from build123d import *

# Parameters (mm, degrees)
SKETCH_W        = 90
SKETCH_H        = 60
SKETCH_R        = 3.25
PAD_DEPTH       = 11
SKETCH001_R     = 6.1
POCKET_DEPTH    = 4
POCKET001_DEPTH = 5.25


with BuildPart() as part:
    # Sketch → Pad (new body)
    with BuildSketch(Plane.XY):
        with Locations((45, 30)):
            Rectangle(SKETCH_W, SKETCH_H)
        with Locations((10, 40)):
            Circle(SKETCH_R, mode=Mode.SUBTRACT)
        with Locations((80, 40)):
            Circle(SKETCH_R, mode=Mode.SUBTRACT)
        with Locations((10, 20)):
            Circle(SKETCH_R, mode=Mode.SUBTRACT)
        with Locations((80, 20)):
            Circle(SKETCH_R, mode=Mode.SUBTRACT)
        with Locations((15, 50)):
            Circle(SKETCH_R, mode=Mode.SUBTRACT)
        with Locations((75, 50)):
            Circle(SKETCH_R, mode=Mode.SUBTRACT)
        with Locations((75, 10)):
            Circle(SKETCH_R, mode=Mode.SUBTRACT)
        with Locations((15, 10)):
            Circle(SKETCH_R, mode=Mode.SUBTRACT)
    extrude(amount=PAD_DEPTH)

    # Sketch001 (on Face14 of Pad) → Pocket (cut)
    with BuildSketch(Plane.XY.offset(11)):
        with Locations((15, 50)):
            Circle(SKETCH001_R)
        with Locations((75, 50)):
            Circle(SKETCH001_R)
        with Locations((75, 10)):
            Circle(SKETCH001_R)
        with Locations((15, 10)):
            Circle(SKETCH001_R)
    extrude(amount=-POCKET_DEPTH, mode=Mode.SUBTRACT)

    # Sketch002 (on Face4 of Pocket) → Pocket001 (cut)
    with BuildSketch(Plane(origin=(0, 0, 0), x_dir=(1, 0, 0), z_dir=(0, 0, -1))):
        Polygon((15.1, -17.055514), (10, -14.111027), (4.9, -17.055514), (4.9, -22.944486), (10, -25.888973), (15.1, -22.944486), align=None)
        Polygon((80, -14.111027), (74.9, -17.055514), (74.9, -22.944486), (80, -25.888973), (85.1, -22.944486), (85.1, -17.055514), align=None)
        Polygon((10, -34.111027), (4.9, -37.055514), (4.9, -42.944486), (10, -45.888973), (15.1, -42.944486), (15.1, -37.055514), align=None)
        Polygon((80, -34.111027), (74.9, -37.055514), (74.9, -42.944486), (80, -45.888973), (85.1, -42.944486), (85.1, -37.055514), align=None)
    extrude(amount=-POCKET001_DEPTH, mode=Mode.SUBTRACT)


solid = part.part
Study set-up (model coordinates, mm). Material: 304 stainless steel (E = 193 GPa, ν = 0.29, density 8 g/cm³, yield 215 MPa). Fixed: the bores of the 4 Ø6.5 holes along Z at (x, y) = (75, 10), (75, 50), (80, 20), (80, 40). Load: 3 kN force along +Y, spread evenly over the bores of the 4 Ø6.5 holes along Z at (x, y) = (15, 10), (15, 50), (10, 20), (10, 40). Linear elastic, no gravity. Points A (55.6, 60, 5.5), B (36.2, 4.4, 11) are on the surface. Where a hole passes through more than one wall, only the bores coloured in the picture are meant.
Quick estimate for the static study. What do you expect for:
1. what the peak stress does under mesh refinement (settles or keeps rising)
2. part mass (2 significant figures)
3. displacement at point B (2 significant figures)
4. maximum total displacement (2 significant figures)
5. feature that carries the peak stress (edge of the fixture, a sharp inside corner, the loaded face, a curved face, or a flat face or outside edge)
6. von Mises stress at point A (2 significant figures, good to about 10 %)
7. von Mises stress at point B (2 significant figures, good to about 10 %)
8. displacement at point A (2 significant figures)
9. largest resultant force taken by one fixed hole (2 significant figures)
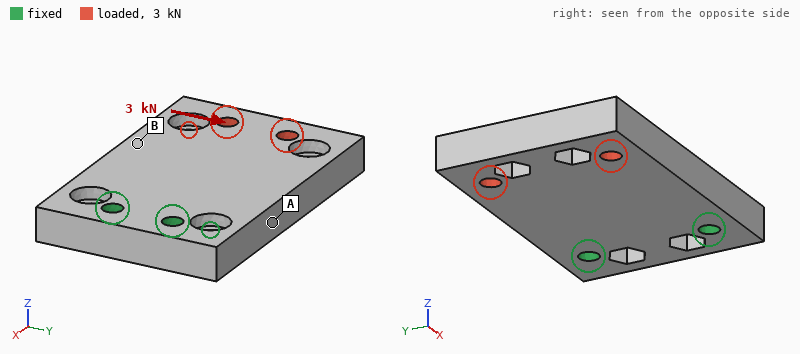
keeps rising
430 g
8.2 µm
17 µm
edge of the fixture
18 MPa
8.1 MPa
5.1 µm
4.1 kN
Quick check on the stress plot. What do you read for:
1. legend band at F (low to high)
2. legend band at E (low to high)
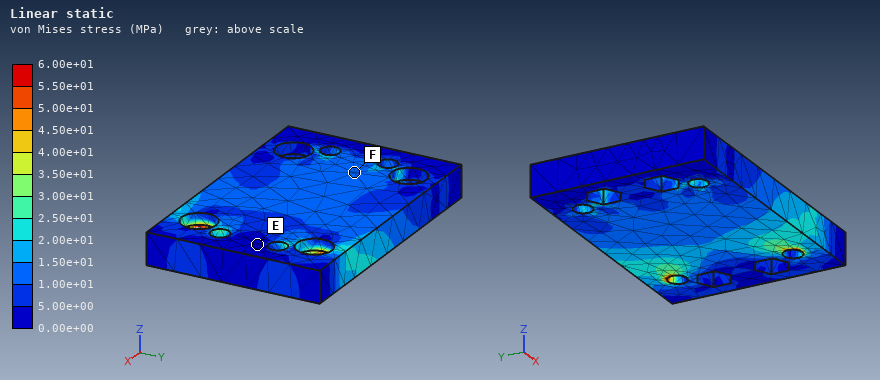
1.00e+01 to 1.50e+01 MPa
0.00e+00 to 5.00e+00 MPa
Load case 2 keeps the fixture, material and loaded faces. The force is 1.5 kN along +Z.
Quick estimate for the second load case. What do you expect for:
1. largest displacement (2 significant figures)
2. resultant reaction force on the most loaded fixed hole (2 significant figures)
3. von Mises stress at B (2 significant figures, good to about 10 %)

0.16 mm
3.2 kN
29 MPa
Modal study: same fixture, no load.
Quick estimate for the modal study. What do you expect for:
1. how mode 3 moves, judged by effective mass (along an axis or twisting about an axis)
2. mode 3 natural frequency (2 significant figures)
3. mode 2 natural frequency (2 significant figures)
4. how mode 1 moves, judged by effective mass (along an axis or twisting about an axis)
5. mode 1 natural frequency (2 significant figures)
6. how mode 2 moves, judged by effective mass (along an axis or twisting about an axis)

along Y
5800 Hz
4000 Hz
along Z
1400 Hz
twisting about X
